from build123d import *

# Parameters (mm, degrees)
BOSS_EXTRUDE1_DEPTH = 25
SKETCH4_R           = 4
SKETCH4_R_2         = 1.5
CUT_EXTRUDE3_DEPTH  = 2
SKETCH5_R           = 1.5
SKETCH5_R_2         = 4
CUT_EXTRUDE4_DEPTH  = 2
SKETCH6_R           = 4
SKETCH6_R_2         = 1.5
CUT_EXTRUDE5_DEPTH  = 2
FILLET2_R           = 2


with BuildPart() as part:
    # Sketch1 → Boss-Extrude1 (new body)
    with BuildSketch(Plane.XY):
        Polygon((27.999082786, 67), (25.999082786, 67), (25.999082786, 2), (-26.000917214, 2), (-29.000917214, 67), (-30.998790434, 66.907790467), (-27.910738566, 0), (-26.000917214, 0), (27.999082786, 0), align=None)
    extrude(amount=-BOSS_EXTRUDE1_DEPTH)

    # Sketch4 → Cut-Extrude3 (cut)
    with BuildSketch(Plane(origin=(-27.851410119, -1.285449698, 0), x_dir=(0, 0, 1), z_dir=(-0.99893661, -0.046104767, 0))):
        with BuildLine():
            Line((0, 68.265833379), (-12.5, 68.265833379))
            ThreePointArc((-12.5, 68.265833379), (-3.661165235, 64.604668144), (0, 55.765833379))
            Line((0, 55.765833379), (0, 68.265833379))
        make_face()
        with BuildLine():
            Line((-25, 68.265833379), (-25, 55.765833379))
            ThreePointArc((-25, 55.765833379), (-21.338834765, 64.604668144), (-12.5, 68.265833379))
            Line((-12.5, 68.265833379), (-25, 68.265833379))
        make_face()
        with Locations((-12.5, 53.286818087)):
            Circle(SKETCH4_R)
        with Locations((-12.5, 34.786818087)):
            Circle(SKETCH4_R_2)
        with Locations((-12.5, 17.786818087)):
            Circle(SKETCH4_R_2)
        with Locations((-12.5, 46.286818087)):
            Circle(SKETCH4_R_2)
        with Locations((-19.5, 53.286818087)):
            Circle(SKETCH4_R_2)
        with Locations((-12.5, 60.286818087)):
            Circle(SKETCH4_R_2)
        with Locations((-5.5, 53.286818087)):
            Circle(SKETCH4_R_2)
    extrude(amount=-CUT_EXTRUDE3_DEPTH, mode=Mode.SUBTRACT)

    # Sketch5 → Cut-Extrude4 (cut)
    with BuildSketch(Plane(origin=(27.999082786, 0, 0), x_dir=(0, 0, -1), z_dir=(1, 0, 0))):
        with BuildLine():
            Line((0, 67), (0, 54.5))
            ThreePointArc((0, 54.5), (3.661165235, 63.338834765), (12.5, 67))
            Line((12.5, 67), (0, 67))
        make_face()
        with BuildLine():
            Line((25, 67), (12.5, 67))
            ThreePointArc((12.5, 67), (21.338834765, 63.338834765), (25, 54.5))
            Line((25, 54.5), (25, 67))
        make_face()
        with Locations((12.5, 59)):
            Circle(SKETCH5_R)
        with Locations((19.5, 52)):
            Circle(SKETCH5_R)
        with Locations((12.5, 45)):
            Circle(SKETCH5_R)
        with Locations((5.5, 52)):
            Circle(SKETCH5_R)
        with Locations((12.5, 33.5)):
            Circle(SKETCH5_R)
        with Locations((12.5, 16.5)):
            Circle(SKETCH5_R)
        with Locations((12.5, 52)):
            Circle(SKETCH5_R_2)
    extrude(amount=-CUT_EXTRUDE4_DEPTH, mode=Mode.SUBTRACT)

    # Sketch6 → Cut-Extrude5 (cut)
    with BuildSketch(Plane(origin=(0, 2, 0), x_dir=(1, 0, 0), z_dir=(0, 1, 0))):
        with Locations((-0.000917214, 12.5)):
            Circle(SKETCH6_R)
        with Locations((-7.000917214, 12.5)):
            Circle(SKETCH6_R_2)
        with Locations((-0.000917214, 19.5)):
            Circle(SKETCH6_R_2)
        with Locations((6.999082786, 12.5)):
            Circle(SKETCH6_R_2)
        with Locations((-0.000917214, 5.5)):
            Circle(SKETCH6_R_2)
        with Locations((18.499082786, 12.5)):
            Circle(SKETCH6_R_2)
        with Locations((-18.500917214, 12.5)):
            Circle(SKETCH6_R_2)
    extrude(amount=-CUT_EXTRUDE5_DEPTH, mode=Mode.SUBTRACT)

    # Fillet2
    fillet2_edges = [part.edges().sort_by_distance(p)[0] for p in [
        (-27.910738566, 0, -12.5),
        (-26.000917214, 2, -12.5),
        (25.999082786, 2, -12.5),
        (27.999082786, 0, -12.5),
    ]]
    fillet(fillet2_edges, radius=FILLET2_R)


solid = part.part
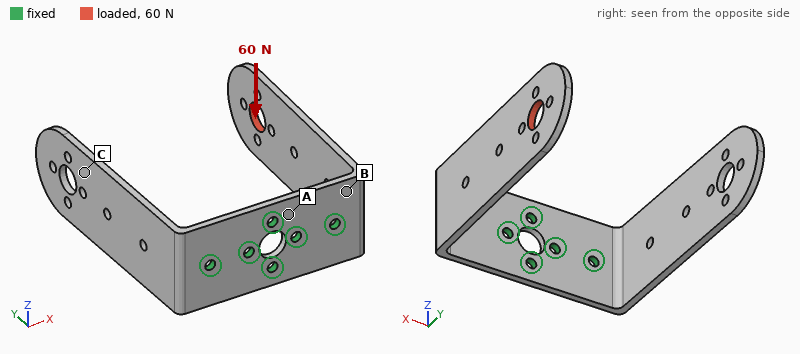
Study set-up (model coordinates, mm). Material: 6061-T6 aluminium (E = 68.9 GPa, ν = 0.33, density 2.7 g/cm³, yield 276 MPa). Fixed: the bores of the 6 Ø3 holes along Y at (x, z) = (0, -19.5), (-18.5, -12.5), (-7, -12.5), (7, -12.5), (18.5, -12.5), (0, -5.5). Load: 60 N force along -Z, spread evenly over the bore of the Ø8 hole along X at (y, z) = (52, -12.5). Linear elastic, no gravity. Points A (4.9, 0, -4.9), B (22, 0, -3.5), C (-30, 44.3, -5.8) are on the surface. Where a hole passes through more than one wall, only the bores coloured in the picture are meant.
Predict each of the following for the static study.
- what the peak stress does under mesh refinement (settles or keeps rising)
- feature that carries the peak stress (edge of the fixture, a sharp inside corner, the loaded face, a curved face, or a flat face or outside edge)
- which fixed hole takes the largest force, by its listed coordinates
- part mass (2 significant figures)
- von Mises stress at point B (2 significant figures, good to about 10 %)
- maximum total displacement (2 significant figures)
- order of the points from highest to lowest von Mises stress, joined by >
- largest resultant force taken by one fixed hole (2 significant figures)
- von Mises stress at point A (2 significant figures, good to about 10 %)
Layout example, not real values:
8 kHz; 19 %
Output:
keeps rising; edge of the fixture; (18.5, -12.5); 23 g; 41 MPa; 0.80 mm; B > A > C; 70 N; 26 MPa
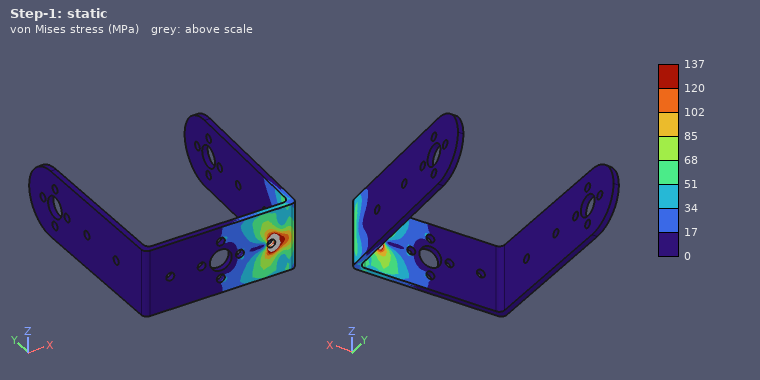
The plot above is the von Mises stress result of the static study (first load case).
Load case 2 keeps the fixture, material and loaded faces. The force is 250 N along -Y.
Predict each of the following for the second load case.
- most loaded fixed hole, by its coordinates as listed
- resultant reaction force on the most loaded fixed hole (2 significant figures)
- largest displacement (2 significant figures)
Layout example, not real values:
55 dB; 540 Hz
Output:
(18.5, -12.5); 310 N; 0.55 mm
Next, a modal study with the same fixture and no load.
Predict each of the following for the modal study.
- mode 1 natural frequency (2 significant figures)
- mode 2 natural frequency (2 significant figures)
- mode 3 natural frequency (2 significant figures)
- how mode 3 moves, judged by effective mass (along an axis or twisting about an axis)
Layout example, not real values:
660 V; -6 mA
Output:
360 Hz; 370 Hz; 770 Hz; along Z
